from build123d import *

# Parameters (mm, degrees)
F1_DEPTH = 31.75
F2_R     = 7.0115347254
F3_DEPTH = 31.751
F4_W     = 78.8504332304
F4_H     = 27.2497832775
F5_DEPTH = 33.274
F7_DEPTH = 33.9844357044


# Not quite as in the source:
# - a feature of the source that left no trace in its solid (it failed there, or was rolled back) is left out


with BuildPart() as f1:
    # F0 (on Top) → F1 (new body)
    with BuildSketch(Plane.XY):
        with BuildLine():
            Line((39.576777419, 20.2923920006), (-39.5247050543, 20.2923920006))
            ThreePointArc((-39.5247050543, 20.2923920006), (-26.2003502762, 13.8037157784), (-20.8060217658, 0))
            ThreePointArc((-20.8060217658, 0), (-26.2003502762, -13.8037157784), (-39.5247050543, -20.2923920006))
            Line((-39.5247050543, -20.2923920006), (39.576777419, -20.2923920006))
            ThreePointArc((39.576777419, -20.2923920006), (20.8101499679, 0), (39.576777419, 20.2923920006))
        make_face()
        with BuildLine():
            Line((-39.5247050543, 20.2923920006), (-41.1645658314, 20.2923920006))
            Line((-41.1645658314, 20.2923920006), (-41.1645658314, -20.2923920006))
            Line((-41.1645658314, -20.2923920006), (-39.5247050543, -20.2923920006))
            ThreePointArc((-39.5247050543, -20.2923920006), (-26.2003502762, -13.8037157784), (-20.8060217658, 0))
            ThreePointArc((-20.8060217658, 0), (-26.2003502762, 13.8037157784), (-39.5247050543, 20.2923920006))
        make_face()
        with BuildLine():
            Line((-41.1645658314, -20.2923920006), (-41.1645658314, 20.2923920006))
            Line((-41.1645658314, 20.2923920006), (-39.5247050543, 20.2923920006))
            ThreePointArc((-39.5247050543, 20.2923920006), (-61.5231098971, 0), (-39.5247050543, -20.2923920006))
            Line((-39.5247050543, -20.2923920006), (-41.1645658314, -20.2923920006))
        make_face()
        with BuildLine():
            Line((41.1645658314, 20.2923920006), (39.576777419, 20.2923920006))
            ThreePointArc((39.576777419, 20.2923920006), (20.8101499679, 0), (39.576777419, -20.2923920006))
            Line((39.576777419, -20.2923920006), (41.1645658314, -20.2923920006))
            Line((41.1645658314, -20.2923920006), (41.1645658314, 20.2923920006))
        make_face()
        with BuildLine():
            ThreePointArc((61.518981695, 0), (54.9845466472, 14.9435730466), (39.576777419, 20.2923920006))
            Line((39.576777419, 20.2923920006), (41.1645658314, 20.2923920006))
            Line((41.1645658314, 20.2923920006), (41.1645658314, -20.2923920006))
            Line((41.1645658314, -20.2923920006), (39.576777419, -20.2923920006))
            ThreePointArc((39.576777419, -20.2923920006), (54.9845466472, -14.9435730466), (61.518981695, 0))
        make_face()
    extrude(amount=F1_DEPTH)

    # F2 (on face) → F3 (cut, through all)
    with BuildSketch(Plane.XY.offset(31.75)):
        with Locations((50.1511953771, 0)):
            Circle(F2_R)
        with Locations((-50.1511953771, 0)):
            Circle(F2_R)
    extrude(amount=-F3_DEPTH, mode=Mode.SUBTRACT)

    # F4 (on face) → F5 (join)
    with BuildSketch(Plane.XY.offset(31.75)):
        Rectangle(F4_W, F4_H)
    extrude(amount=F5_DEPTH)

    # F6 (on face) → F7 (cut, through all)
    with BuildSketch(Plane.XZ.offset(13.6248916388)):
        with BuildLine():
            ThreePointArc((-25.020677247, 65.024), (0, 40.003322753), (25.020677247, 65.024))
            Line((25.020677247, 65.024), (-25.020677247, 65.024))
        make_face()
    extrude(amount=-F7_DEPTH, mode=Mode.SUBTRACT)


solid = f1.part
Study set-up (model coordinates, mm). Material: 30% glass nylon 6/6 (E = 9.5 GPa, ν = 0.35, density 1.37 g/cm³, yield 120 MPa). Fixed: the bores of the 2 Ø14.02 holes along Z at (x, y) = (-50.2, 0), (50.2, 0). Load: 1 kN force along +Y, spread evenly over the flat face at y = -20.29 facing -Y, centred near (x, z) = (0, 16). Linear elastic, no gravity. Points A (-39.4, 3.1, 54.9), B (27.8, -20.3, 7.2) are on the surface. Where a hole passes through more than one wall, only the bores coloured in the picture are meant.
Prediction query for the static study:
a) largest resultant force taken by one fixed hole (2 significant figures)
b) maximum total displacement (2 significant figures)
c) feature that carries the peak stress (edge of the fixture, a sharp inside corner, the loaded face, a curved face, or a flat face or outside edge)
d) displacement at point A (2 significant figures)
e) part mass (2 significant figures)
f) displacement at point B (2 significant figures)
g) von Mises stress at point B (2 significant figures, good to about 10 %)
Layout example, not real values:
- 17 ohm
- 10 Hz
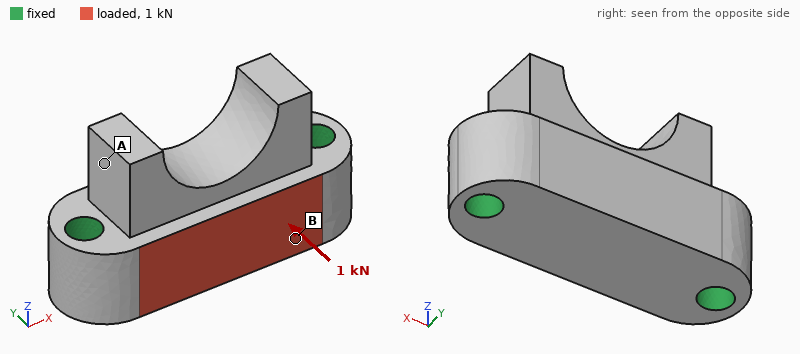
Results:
- 510 N
- 7.3 µm
- edge of the fixture
- 2.8 µm
- 250 g
- 4.7 µm
- 0.48 MPa
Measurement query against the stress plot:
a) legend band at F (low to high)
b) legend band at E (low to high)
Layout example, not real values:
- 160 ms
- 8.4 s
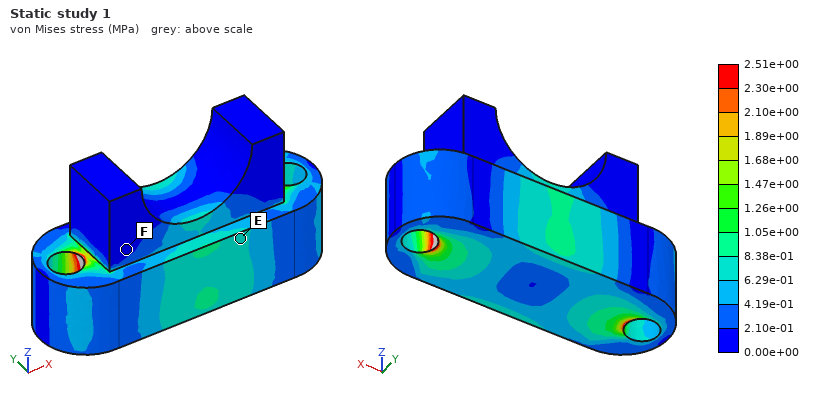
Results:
- 0.00e+00 to 2.10e-01 MPa
- 6.29e-01 to 8.38e-01 MPa
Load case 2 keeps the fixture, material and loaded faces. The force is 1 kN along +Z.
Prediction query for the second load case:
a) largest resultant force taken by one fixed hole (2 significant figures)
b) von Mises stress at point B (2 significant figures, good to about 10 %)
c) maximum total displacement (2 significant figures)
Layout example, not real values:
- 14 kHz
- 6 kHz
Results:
- 510 N
- 1.5 MPa
- 15 µm
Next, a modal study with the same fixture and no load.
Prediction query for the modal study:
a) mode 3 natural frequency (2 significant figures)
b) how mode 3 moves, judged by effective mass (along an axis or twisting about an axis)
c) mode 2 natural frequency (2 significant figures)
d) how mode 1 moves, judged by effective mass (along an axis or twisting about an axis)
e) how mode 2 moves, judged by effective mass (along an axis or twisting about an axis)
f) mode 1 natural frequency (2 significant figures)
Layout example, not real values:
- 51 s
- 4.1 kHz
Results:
- 5800 Hz
- along Y
- 5300 Hz
- along Y
- along Z
- 4000 Hz
